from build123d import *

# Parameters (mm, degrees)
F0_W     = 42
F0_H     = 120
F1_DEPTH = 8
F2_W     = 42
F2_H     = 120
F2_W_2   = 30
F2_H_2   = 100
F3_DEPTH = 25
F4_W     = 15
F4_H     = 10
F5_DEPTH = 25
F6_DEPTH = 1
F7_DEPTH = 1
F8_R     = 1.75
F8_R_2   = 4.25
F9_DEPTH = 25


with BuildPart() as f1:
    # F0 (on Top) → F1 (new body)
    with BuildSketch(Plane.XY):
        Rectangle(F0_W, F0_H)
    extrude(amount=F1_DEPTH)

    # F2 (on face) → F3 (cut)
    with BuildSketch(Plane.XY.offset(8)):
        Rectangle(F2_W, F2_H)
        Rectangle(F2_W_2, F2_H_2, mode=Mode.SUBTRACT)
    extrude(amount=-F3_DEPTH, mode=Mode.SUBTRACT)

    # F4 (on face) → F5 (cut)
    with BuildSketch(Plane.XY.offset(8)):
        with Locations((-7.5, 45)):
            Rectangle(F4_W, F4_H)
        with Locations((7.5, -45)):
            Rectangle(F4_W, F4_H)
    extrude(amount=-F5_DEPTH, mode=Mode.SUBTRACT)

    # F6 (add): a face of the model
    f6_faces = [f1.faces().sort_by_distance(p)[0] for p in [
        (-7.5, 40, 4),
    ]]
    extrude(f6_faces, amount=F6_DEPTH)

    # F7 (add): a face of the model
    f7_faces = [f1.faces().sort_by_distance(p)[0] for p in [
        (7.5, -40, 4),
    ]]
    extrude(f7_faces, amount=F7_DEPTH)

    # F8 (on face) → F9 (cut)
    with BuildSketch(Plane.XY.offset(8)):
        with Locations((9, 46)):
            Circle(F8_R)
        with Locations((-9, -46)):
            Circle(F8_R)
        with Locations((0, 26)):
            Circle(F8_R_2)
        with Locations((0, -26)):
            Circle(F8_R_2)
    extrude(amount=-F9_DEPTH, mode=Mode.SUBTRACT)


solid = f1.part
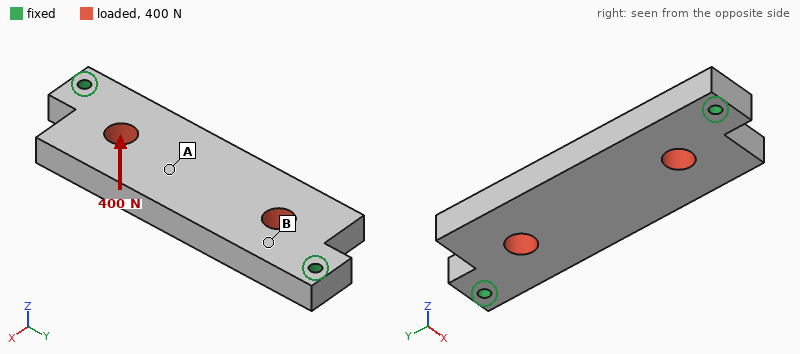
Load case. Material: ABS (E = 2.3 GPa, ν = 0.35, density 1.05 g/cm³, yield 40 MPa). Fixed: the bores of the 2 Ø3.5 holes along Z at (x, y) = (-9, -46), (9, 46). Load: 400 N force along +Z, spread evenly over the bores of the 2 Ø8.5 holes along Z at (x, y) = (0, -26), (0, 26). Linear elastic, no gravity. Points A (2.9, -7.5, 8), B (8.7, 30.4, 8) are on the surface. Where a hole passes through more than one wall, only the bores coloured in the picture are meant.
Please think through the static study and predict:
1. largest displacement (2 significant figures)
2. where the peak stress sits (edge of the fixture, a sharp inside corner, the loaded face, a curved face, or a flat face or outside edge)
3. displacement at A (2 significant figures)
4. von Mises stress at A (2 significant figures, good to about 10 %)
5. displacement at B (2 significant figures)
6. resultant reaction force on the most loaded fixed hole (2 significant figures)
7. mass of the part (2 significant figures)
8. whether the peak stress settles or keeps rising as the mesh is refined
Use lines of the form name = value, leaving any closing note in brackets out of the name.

largest displacement = 0.47 mm
where the peak stress sits = edge of the fixture
displacement at A = 0.44 mm
von Mises stress at A = 4.3 MPa
displacement at B = 0.20 mm
resultant reaction force on the most loaded fixed hole = 200 N
mass of the part = 22 g
whether the peak stress settles or keeps rising as the mesh is refined = keeps rising
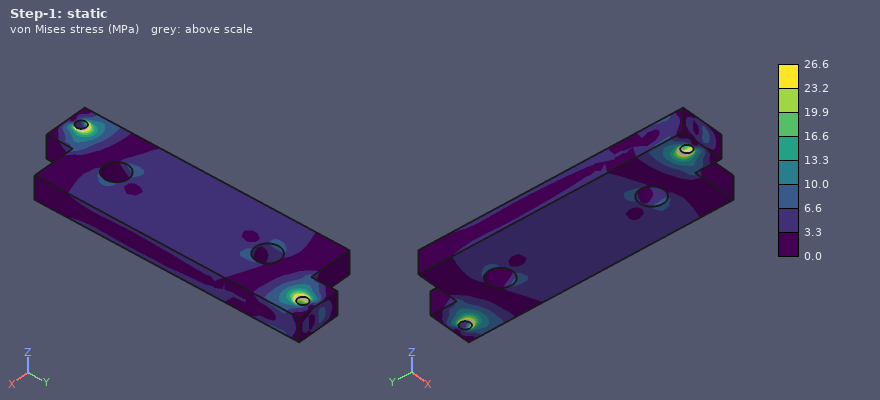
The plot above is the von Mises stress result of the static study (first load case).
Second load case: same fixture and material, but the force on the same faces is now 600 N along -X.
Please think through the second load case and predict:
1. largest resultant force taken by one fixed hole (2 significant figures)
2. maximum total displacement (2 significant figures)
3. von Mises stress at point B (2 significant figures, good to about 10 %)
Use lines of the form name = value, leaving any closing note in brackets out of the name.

largest resultant force taken by one fixed hole = 300 N
maximum total displacement = 0.18 mm
von Mises stress at point B = 2.3 MPa
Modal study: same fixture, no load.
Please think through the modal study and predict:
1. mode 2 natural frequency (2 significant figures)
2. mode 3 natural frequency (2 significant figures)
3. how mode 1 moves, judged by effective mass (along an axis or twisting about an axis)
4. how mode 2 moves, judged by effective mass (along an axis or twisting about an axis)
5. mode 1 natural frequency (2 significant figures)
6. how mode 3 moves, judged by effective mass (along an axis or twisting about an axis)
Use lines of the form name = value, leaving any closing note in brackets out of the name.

mode 2 natural frequency = 1500 Hz
mode 3 natural frequency = 2000 Hz
how mode 1 moves, judged by effective mass = along Z
how mode 2 moves, judged by effective mass = twisting about Y
mode 1 natural frequency = 1100 Hz
how mode 3 moves, judged by effective mass = along X
